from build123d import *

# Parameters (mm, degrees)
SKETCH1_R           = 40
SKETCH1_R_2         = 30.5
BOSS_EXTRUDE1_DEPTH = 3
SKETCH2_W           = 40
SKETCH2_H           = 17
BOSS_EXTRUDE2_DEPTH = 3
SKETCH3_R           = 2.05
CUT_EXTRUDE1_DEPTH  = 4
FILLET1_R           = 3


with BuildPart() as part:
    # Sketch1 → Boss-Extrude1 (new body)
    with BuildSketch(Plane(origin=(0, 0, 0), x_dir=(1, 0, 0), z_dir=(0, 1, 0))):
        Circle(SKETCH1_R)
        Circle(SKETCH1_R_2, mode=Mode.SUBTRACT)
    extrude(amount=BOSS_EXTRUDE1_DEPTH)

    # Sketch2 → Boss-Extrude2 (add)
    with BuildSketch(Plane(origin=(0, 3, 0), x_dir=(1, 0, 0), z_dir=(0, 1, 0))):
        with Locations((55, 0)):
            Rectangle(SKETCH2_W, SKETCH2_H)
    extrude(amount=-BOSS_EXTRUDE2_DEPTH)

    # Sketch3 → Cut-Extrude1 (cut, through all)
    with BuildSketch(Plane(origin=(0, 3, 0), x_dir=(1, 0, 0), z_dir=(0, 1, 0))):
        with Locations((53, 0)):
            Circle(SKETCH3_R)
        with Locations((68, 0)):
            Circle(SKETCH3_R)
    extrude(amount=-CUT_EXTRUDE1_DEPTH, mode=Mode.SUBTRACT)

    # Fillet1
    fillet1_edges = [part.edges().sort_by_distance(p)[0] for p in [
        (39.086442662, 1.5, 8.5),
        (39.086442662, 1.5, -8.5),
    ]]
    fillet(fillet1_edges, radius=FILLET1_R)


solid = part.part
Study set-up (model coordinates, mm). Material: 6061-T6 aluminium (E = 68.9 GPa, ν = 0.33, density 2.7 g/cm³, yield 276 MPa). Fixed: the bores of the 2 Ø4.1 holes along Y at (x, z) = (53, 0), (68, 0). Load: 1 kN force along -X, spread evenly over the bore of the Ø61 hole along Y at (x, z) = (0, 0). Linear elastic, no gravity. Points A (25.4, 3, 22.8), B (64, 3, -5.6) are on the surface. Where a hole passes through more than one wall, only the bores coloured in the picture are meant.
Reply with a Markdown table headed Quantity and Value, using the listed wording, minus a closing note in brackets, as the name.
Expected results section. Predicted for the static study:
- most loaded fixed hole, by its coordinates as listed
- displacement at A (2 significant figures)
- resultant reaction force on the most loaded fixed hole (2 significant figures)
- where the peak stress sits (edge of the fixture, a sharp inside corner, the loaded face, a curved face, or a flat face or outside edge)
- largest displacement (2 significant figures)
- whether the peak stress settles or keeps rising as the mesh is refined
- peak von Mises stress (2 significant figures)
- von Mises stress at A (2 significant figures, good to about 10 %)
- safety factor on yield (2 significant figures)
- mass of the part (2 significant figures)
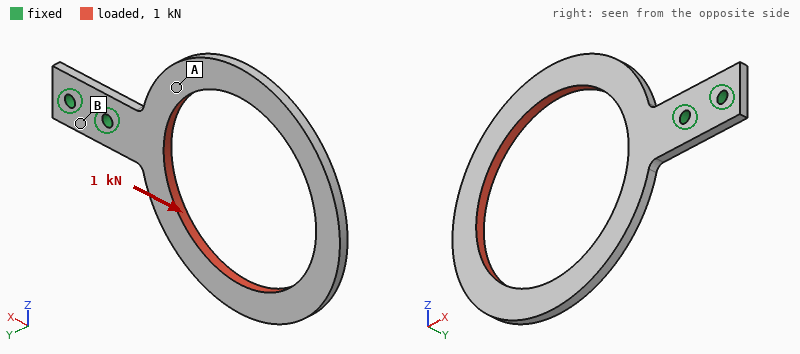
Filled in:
| Quantity | Value |
|---|---|
| most loaded fixed hole, by its coordinates as listed | (53, 0) |
| displacement at A | 0.079 mm |
| resultant reaction force on the most loaded fixed hole | 860 N |
| where the peak stress sits | a curved face |
| largest displacement | 0.20 mm |
| whether the peak stress settles or keeps rising as the mesh is refined | settles |
| peak von Mises stress | 200 MPa |
| von Mises stress at A | 26 MPa |
| safety factor on yield | 1.4 |
| mass of the part | 22 g |
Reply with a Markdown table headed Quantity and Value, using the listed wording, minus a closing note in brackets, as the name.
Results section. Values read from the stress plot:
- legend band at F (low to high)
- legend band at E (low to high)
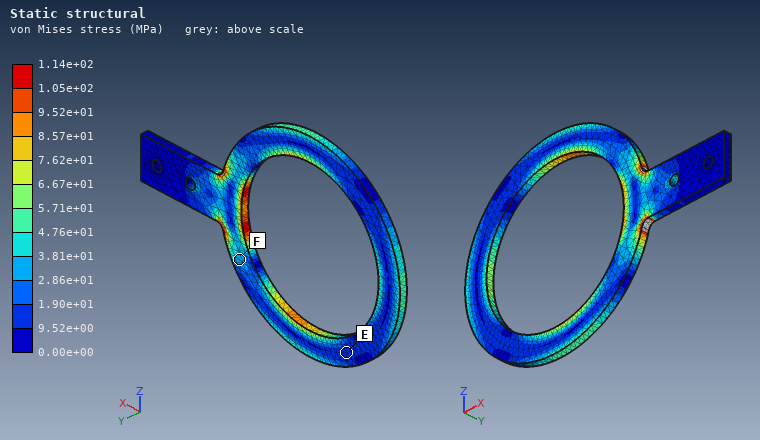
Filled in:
| Quantity | Value |
|---|---|
| legend band at F | 2.86e+01 to 3.81e+01 MPa |
| legend band at E | 9.52e+00 to 1.90e+01 MPa |
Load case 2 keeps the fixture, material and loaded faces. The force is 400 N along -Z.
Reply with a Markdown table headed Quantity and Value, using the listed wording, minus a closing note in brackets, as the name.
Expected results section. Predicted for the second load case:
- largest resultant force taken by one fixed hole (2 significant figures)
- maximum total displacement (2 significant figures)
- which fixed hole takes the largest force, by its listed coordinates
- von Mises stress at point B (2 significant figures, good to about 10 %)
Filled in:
| Quantity | Value |
|---|---|
| largest resultant force taken by one fixed hole | 1.3 kN |
| maximum total displacement | 1.0 mm |
| which fixed hole takes the largest force, by its listed coordinates | (53, 0) |
| von Mises stress at point B | 36 MPa |
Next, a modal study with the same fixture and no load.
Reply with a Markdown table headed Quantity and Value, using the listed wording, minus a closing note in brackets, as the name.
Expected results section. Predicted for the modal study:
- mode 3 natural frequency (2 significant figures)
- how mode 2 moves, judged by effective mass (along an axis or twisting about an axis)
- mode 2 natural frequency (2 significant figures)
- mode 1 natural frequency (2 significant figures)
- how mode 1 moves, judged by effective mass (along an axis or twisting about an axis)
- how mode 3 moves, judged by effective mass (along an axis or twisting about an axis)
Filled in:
| Quantity | Value |
|---|---|
| mode 3 natural frequency | 830 Hz |
| how mode 2 moves, judged by effective mass | twisting about X |
| mode 2 natural frequency | 460 Hz |
| mode 1 natural frequency | 210 Hz |
| how mode 1 moves, judged by effective mass | along Y |
| how mode 3 moves, judged by effective mass | along Z |
